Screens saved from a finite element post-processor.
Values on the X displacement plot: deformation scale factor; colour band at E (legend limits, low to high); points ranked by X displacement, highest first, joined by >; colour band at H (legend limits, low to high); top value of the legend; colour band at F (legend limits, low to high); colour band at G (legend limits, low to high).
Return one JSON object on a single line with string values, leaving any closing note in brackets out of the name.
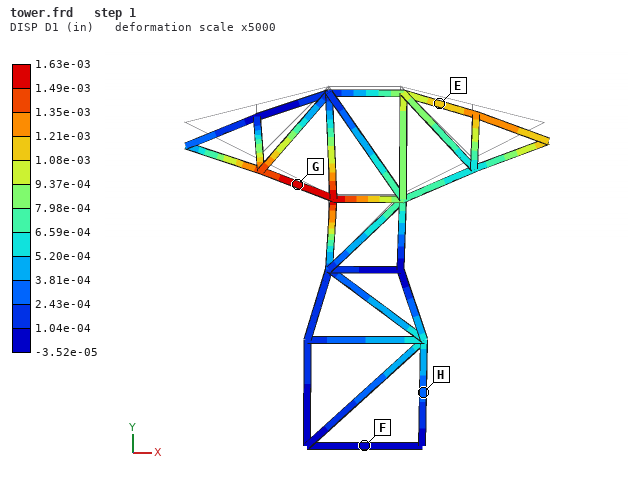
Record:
{"deformation scale factor": "5000", "colour band at E": "1.08e-03 to 1.21e-03 in", "points ranked by X displacement, highest first, joined by >": "G > E > H > F", "colour band at H": "2.43e-04 to 3.81e-04 in", "top value of the legend": "1.63e-03 in", "colour band at F": "-3.52e-05 to 1.04e-04 in", "colour band at G": "1.49e-03 to 1.63e-03 in"}
